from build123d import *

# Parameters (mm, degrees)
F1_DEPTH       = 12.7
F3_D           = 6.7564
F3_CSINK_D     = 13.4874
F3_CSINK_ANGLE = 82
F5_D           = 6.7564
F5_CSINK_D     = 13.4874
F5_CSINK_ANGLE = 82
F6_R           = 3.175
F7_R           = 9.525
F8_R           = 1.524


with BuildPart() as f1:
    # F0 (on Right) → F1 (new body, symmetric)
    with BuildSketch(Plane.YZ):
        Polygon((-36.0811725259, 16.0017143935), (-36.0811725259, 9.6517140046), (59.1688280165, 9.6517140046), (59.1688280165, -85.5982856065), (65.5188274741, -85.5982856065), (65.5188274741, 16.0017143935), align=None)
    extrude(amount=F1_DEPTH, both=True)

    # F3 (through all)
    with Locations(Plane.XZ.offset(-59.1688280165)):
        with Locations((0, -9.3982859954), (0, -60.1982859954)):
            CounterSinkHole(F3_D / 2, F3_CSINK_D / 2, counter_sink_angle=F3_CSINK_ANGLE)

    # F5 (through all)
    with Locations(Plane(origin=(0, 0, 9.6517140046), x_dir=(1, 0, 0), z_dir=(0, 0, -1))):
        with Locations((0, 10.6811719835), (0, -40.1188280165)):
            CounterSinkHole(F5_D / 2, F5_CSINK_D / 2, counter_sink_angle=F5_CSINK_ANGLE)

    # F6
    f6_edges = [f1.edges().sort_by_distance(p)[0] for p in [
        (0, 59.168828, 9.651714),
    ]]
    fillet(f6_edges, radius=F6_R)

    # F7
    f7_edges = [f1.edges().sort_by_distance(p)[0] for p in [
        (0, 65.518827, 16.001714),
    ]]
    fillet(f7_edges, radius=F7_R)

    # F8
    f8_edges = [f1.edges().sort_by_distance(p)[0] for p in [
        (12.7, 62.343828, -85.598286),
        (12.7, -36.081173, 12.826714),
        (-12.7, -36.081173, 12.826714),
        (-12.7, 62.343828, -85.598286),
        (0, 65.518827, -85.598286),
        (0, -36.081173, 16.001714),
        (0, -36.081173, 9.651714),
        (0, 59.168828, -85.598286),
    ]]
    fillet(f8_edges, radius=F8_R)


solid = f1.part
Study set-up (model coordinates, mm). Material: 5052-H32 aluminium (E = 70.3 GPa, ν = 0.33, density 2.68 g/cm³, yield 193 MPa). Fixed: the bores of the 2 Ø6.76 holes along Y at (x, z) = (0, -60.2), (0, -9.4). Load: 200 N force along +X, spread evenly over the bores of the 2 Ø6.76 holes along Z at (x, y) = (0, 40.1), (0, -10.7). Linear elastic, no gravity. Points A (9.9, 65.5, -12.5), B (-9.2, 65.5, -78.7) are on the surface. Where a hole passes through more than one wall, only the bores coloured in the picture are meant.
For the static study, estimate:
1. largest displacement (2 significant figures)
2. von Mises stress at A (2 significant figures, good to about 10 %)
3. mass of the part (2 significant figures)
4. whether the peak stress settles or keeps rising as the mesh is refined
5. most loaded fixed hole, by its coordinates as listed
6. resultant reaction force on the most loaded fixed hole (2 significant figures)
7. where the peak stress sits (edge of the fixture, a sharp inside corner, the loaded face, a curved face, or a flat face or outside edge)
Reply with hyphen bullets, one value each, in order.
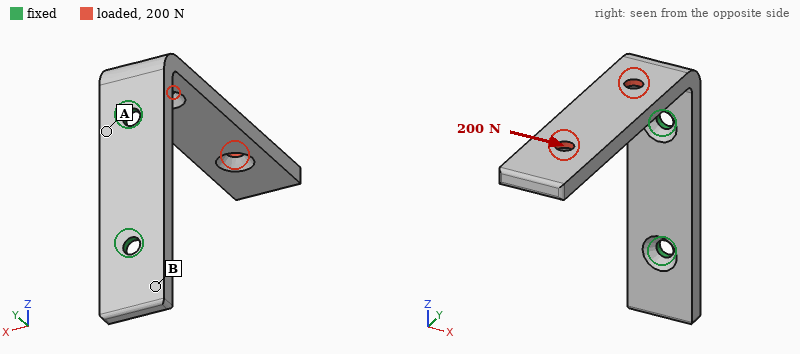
- 0.55 mm
- 34 MPa
- 79 g
- keeps rising
- (0, -9.4)
- 240 N
- edge of the fixture
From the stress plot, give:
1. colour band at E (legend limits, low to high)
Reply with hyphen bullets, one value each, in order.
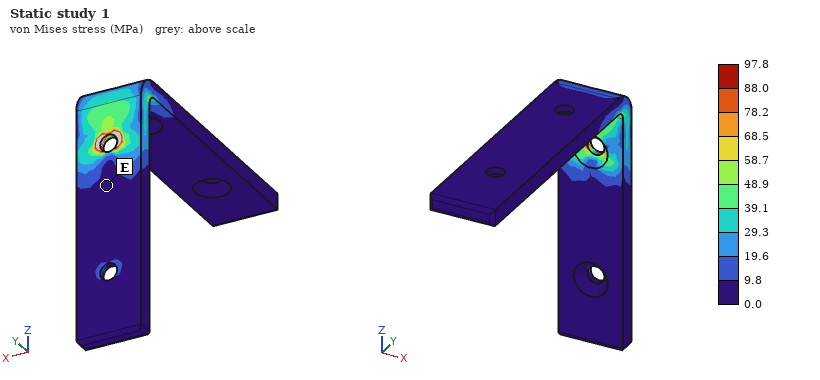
- 0.0 to 9.8 MPa
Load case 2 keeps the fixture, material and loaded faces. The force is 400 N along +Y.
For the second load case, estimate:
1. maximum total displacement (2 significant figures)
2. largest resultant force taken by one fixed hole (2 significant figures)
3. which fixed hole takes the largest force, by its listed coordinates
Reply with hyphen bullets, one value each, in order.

- 0.50 mm
- 610 N
- (0, -9.4)
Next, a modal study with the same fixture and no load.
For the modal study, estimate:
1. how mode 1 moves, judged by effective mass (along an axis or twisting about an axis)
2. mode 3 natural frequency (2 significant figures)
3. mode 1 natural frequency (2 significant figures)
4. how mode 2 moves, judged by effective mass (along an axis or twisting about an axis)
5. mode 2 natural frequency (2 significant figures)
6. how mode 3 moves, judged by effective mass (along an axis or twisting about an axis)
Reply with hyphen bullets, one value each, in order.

- along Z
- 2100 Hz
- 380 Hz
- along X
- 570 Hz
- along Y
